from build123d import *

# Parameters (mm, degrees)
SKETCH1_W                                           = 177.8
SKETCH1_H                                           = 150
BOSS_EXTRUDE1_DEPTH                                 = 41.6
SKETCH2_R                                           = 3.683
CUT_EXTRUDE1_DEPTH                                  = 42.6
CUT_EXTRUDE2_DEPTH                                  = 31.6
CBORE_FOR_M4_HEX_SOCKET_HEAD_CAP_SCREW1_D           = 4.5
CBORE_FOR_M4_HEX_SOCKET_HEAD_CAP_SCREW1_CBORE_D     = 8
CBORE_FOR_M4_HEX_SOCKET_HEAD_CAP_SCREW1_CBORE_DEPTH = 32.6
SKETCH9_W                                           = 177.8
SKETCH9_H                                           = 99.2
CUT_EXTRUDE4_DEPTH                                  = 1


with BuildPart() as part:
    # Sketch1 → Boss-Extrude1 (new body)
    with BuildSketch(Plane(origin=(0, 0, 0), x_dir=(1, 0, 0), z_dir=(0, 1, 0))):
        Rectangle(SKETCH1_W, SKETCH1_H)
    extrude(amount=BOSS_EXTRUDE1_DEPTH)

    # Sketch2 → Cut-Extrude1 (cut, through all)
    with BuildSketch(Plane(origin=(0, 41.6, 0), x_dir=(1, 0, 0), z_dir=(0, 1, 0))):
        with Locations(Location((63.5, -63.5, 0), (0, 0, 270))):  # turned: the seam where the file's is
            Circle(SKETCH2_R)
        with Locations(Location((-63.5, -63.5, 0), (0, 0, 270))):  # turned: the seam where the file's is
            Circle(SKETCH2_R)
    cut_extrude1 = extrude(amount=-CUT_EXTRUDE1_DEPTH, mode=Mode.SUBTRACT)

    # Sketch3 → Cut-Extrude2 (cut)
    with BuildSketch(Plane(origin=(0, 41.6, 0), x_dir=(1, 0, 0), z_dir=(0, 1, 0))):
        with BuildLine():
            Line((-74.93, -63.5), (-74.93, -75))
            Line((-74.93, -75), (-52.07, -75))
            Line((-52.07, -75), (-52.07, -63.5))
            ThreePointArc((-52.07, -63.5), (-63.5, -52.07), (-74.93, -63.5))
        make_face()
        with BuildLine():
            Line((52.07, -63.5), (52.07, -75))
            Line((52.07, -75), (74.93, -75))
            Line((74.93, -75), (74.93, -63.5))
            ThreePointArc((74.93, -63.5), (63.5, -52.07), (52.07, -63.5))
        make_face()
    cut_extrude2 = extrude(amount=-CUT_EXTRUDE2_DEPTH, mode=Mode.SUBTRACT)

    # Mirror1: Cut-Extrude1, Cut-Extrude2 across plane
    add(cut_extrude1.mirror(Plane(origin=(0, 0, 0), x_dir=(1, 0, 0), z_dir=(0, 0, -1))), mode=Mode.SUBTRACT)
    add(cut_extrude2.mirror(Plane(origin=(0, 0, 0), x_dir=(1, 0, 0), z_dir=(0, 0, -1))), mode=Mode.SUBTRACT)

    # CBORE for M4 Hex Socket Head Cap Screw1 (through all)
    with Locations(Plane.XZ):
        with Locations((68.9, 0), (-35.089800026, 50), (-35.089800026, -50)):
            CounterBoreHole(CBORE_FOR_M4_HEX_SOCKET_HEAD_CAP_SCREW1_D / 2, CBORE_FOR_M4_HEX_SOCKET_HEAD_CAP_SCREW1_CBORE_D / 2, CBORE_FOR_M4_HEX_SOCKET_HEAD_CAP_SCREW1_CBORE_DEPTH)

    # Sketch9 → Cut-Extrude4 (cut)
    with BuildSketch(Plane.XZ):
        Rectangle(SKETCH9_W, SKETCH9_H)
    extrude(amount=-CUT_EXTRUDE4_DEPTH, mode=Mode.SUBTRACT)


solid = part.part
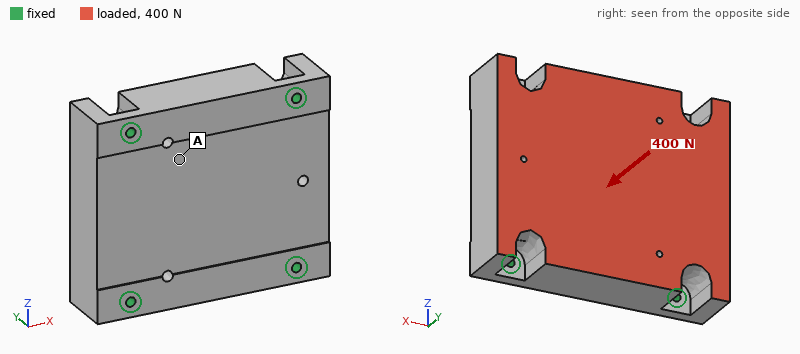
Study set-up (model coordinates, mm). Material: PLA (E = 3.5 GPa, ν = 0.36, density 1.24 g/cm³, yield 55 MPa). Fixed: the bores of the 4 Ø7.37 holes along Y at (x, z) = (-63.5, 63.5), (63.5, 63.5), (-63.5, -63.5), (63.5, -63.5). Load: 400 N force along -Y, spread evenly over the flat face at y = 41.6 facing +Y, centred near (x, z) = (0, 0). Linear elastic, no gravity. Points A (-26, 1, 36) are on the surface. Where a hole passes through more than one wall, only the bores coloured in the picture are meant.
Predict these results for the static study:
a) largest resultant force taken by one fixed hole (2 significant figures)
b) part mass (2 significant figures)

110 N
1.3 kg
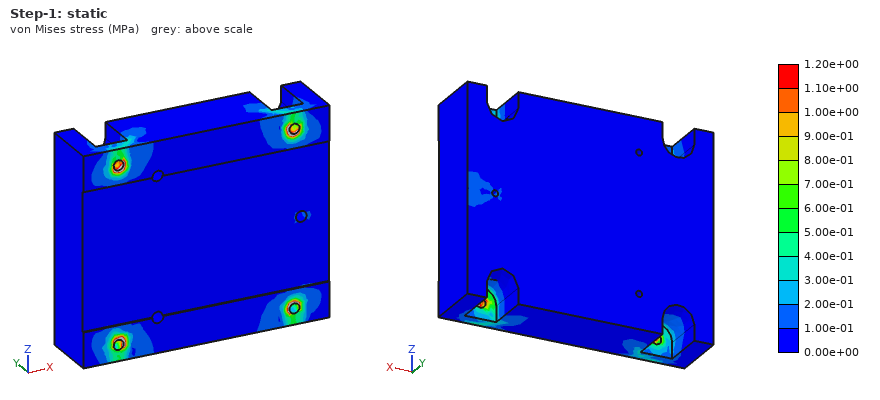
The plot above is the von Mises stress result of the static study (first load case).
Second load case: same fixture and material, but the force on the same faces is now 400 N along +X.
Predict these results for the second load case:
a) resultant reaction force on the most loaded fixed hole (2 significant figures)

120 N
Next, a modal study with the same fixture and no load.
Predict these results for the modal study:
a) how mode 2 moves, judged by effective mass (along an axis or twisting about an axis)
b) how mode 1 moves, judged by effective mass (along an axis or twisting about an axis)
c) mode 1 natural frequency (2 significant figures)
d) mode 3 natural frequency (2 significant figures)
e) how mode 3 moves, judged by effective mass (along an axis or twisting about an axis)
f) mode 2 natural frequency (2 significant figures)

along X
along Y
1200 Hz
1600 Hz
along Z
1400 Hz
